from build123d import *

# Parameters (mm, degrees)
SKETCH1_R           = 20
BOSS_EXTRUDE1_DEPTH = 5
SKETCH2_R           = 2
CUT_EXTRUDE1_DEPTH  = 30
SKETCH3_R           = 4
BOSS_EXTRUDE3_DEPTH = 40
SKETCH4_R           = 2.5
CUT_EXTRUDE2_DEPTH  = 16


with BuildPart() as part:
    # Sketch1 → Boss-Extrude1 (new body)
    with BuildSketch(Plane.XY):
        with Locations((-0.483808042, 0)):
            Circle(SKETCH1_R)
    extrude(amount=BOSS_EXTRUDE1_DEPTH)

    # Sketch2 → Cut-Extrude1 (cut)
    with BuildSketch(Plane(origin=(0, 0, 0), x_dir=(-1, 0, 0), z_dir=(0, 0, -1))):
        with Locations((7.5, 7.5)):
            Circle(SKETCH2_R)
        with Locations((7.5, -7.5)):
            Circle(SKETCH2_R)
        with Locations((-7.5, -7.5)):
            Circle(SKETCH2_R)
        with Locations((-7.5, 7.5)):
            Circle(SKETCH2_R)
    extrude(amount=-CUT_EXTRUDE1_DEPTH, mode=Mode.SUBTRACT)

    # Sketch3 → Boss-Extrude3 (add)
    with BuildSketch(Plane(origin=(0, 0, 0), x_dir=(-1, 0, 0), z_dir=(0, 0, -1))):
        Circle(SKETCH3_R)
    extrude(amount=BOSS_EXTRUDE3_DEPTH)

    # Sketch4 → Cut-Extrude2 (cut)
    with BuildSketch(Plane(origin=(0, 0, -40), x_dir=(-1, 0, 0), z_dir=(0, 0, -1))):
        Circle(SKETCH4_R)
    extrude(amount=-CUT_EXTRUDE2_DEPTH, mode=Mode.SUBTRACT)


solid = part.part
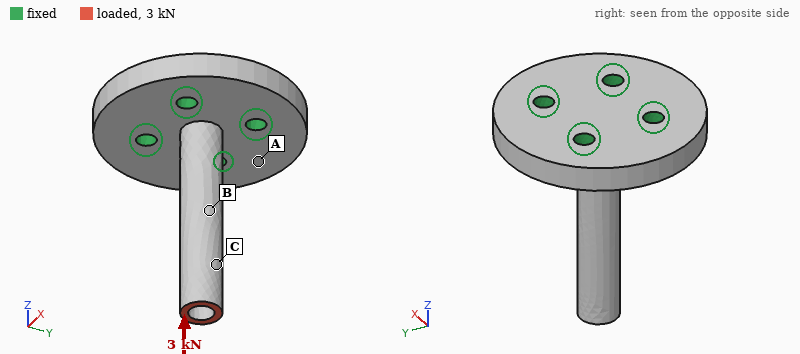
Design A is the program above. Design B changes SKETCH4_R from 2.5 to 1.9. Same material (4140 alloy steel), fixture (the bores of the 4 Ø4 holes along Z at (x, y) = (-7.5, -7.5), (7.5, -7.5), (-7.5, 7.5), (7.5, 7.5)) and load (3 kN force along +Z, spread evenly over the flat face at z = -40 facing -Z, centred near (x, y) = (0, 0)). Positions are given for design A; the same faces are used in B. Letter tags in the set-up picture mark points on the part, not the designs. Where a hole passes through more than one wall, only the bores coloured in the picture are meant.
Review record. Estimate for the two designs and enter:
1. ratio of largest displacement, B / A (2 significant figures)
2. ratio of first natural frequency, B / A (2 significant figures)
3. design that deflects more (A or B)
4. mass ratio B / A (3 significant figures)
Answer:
0.90
0.91
A
1.02
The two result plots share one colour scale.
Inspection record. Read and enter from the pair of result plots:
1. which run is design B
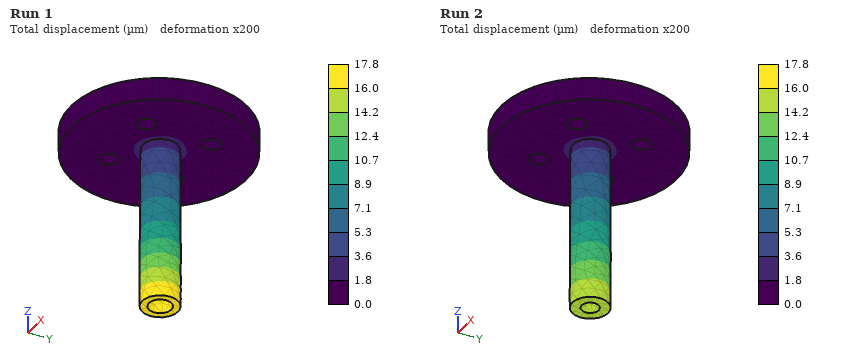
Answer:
Run 2
